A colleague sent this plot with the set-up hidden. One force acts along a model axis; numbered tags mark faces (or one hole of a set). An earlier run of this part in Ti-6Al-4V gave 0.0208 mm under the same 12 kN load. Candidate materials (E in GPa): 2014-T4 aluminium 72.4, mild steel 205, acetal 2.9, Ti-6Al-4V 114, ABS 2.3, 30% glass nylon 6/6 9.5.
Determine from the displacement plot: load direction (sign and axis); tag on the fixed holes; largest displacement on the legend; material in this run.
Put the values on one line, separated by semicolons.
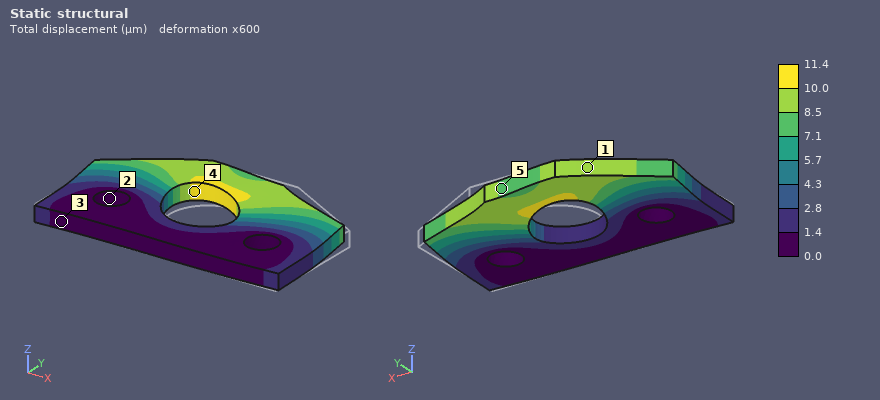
-X; 2; 11.4 µm; mild steel
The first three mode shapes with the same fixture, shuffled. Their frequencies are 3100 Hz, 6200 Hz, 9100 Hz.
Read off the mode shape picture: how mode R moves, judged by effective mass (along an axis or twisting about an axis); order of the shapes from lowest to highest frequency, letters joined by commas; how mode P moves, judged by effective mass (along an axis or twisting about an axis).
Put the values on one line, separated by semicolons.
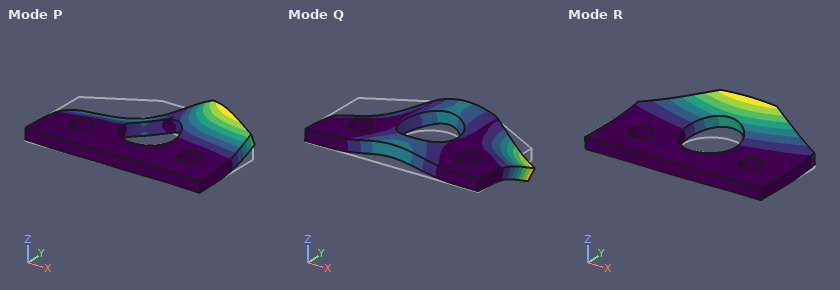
along Z; R, P, Q; twisting about Y
